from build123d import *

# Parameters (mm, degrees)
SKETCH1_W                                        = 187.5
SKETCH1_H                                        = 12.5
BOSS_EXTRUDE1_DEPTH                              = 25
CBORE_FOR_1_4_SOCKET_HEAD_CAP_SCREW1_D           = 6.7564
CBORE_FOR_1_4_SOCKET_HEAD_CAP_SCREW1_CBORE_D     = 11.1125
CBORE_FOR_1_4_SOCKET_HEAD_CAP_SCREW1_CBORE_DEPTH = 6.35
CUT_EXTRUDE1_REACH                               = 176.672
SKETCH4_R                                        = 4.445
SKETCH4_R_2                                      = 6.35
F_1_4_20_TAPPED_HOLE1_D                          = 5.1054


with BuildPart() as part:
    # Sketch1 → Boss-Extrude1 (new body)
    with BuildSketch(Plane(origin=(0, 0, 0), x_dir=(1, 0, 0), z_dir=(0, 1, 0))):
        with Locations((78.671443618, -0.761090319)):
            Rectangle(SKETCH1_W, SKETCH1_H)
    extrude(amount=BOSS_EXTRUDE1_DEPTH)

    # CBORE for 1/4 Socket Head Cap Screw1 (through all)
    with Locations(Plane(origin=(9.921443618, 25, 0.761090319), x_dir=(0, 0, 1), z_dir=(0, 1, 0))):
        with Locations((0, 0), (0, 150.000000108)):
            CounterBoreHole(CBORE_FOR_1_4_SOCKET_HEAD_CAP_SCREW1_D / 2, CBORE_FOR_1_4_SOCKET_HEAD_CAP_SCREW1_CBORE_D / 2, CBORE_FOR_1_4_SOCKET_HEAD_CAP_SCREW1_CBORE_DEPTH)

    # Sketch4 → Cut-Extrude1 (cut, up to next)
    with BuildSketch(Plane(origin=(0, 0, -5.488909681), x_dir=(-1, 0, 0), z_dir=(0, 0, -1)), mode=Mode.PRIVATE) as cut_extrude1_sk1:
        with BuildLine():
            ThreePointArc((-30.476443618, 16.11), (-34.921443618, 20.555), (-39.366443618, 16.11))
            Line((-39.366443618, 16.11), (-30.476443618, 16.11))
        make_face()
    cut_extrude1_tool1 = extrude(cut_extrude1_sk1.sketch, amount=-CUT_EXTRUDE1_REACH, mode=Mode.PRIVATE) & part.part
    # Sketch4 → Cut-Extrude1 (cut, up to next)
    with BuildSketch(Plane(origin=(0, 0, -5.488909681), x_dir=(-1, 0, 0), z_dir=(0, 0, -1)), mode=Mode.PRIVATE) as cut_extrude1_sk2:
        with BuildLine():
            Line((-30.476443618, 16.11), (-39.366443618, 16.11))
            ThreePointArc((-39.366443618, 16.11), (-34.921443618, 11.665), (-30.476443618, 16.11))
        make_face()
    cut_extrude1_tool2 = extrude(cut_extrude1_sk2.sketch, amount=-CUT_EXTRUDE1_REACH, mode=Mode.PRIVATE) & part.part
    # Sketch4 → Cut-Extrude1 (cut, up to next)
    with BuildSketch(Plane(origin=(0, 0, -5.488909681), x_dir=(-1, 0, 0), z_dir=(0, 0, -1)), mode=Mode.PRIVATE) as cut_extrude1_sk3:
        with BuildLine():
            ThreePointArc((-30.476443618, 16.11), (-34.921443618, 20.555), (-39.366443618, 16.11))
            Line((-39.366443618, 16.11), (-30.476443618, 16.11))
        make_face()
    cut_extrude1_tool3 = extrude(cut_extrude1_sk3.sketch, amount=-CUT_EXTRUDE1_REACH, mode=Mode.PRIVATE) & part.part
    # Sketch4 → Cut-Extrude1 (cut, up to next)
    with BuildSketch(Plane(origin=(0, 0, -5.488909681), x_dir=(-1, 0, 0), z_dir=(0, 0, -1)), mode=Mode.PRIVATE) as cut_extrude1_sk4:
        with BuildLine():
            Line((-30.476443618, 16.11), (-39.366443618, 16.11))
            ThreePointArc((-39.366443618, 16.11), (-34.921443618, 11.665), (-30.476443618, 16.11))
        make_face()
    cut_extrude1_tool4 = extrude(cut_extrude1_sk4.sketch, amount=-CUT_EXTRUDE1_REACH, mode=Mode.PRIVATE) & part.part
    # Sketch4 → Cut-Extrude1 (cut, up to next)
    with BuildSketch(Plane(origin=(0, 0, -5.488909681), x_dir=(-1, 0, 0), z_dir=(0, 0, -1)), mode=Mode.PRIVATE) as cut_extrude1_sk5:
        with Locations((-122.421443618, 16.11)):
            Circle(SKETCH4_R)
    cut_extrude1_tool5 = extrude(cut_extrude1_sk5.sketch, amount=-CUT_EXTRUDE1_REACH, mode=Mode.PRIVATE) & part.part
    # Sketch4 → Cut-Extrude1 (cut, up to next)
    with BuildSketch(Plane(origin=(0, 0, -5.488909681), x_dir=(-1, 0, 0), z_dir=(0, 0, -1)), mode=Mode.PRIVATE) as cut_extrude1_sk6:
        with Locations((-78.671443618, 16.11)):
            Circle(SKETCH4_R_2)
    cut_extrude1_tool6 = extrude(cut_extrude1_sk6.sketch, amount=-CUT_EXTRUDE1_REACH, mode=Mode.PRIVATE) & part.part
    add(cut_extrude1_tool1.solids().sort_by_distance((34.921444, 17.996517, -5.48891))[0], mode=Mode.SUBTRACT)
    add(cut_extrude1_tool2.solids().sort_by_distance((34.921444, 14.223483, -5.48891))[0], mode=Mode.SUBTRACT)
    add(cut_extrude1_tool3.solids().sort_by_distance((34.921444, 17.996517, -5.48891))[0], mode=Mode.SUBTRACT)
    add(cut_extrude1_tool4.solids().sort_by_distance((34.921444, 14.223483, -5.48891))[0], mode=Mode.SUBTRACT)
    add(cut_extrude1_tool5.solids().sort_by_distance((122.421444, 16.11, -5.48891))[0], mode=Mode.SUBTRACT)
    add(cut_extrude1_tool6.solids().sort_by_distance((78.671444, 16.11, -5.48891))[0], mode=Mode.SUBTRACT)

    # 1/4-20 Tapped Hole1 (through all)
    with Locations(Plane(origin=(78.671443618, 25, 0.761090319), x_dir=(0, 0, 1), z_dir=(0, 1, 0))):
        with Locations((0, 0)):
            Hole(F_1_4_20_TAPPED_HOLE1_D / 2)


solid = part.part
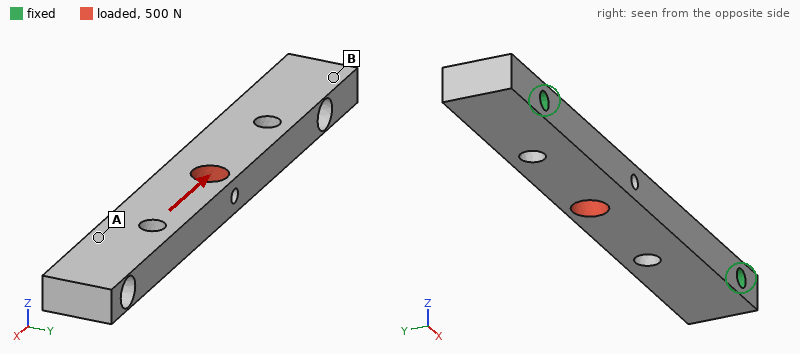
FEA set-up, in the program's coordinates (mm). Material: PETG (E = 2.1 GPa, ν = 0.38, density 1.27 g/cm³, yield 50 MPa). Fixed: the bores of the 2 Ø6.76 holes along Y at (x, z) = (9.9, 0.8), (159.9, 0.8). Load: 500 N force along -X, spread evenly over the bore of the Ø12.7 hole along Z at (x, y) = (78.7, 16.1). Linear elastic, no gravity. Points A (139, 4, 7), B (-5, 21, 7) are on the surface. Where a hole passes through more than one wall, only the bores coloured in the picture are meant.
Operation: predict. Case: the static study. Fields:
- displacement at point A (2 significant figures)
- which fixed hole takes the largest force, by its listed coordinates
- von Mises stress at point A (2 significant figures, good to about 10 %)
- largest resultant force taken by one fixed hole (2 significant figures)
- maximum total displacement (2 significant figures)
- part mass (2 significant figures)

9.8 µm
(9.9, 0.8)
0.94 MPa
270 N
38 µm
67 g
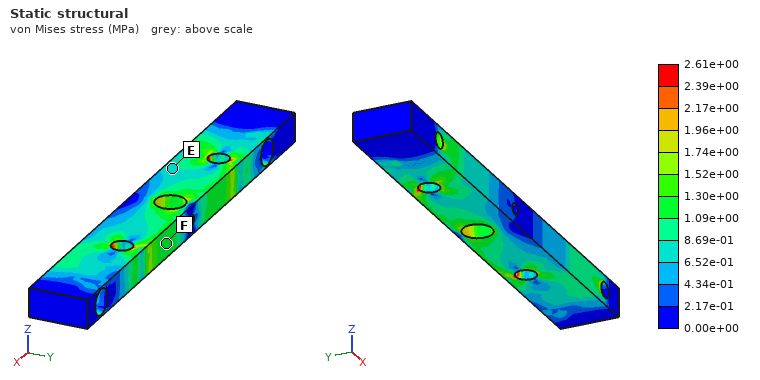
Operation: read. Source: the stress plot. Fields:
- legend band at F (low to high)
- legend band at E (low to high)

1.09e+00 to 1.30e+00 MPa
6.52e-01 to 8.69e-01 MPa
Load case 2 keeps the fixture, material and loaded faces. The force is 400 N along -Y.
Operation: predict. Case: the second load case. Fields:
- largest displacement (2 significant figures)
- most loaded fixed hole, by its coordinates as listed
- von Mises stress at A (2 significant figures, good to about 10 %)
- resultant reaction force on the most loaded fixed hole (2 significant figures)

0.38 mm
(9.9, 0.8)
2.0 MPa
220 N
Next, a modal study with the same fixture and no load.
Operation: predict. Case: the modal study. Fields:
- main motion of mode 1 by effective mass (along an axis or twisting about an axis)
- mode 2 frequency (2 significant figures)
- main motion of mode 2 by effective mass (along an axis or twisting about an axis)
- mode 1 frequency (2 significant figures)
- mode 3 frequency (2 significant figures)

along Z
1100 Hz
along Y
670 Hz
1700 Hz
